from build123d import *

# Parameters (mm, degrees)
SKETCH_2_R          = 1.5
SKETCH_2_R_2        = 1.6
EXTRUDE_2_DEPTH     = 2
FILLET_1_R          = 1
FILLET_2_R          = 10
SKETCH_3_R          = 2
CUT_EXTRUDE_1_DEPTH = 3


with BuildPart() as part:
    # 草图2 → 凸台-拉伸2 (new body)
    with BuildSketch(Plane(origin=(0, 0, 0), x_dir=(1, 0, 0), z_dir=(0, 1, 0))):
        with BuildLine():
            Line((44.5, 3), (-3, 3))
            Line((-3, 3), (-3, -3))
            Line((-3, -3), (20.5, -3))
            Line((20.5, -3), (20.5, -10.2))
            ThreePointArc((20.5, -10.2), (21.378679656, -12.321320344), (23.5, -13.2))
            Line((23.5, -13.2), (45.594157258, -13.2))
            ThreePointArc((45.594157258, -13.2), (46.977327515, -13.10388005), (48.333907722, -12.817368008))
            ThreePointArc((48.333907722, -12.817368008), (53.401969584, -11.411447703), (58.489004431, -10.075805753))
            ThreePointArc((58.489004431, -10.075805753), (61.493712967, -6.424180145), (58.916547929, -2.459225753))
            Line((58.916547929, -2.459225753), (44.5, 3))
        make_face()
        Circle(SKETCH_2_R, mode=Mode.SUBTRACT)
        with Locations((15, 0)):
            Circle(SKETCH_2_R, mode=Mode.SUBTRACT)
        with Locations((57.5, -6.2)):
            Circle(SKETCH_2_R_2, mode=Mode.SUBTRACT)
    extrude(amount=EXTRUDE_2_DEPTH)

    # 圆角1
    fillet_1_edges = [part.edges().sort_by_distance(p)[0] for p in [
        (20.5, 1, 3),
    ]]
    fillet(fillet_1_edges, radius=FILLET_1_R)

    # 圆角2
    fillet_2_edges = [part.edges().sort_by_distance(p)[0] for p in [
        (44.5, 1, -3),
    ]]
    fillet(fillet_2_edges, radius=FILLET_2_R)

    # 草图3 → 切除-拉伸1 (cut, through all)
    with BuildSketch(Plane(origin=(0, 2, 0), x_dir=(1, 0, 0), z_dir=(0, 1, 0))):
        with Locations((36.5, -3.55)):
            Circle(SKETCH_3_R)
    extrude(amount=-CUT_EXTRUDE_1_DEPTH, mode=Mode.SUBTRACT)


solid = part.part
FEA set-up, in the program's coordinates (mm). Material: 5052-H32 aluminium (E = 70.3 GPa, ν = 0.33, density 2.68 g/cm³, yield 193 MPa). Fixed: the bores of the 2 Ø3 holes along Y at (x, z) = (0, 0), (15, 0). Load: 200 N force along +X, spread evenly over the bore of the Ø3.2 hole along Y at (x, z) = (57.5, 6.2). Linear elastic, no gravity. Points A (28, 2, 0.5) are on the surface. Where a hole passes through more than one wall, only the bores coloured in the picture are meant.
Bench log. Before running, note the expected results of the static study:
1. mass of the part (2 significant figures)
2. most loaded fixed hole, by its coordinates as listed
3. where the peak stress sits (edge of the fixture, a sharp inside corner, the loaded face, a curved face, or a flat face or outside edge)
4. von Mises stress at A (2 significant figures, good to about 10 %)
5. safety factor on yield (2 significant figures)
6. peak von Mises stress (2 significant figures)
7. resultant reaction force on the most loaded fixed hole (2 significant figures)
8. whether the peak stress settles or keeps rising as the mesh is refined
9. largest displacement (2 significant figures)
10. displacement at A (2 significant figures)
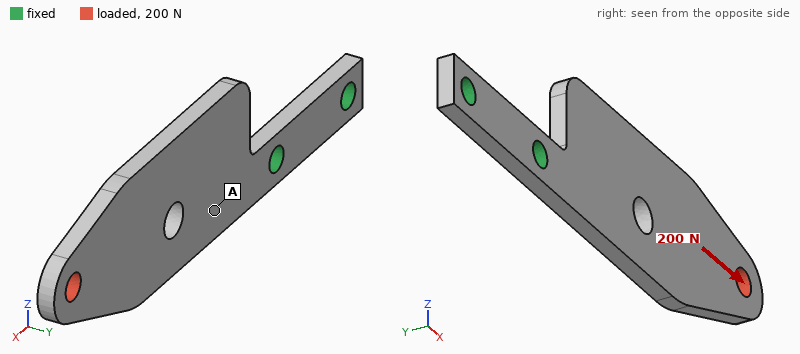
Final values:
3.7 g
(15, 0)
a curved face
12 MPa
0.86
220 MPa
200 N
settles
0.18 mm
0.038 mm
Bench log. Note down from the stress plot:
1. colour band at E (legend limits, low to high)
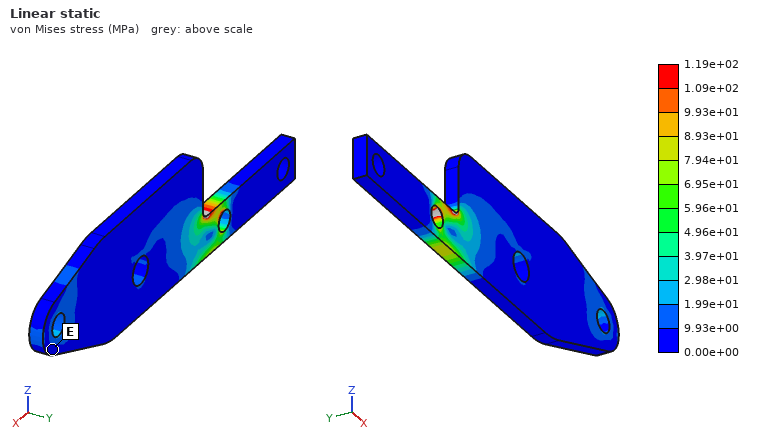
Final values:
0.00e+00 to 9.93e+00 MPa
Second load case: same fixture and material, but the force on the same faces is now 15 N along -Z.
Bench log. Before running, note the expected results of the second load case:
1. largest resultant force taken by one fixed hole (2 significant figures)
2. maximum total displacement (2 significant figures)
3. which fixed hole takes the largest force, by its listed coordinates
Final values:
22 N
92 µm
(15, 0)
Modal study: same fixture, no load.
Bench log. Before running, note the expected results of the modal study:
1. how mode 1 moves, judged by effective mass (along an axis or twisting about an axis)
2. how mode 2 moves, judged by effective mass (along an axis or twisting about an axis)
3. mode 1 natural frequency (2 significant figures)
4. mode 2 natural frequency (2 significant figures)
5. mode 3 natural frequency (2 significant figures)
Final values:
along Y
along Z
710 Hz
2100 Hz
3400 Hz
